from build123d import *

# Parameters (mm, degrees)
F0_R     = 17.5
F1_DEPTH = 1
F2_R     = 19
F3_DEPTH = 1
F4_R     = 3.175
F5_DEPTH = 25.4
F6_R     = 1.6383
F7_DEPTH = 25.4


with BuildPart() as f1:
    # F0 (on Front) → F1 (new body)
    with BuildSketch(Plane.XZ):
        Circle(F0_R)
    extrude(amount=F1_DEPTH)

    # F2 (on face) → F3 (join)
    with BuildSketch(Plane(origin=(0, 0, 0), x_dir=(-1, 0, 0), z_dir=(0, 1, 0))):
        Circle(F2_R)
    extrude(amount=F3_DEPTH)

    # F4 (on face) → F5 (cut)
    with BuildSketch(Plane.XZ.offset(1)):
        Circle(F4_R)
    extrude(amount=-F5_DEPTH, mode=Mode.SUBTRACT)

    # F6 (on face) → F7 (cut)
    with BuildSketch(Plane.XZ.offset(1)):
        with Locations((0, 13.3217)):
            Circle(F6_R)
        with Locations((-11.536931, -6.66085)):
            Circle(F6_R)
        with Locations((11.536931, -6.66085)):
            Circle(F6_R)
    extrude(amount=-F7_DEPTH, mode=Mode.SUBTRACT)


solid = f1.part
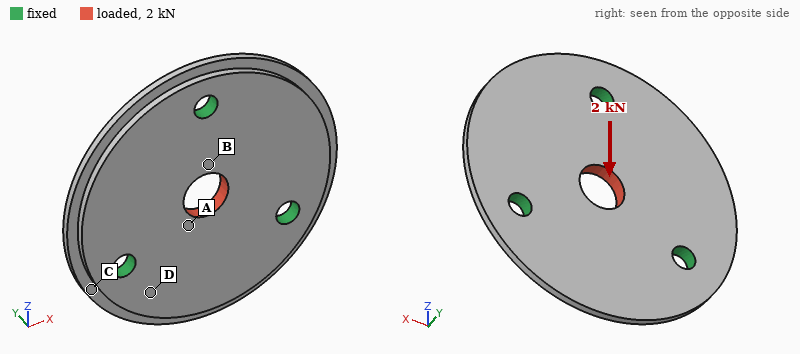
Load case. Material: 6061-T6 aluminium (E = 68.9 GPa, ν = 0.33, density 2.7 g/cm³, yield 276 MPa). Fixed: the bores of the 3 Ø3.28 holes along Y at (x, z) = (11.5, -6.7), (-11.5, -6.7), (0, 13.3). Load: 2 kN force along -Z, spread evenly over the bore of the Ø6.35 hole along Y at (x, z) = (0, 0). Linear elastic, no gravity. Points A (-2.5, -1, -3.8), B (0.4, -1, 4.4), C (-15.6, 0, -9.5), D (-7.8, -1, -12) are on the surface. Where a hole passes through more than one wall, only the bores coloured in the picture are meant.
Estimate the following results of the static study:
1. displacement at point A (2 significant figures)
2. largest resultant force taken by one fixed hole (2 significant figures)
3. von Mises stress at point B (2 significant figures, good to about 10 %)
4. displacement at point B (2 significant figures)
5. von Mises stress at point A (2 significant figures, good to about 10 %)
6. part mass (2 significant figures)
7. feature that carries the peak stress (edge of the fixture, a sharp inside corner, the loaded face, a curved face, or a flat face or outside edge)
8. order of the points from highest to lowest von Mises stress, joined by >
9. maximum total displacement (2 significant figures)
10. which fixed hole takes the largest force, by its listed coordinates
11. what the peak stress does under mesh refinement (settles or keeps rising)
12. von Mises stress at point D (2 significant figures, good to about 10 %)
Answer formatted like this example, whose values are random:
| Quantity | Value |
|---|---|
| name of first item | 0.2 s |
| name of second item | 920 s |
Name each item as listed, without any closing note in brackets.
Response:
| Quantity | Value |
|---|---|
| displacement at point A | 7.8 µm |
| largest resultant force taken by one fixed hole | 720 N |
| von Mises stress at point B | 56 MPa |
| displacement at point B | 5.6 µm |
| von Mises stress at point A | 40 MPa |
| part mass | 5.4 g |
| feature that carries the peak stress | edge of the fixture |
| order of the points from highest to lowest von Mises stress, joined by > | B > A > D > C |
| maximum total displacement | 9.6 µm |
| which fixed hole takes the largest force, by its listed coordinates | (0, 13.3) |
| what the peak stress does under mesh refinement | keeps rising |
| von Mises stress at point D | 21 MPa |
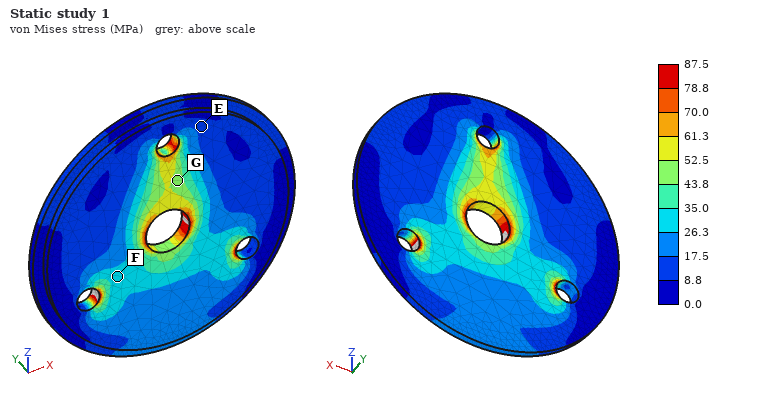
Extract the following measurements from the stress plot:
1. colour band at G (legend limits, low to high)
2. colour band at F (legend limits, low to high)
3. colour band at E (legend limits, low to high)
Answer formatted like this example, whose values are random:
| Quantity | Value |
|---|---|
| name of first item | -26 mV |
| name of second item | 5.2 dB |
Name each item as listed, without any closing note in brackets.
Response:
| Quantity | Value |
|---|---|
| colour band at G | 43.8 to 52.5 MPa |
| colour band at F | 26.3 to 35.0 MPa |
| colour band at E | 8.8 to 17.5 MPa |
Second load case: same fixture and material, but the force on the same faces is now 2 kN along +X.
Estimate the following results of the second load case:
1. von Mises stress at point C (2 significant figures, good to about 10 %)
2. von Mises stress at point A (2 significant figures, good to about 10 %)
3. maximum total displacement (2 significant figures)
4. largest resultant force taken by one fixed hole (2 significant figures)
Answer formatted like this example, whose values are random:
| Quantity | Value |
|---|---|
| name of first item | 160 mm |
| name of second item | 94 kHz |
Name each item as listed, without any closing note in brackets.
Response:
| Quantity | Value |
|---|---|
| von Mises stress at point C | 11 MPa |
| von Mises stress at point A | 52 MPa |
| maximum total displacement | 9.3 µm |
| largest resultant force taken by one fixed hole | 700 N |
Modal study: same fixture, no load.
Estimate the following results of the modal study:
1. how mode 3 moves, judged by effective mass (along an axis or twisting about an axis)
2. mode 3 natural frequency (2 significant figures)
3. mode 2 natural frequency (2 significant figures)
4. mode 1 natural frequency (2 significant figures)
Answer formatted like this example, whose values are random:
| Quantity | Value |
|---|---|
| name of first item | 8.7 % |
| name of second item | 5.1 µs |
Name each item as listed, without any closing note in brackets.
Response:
| Quantity | Value |
|---|---|
| how mode 3 moves, judged by effective mass | along Y |
| mode 3 natural frequency | 13 kHz |
| mode 2 natural frequency | 12 kHz |
| mode 1 natural frequency | 12 kHz |
